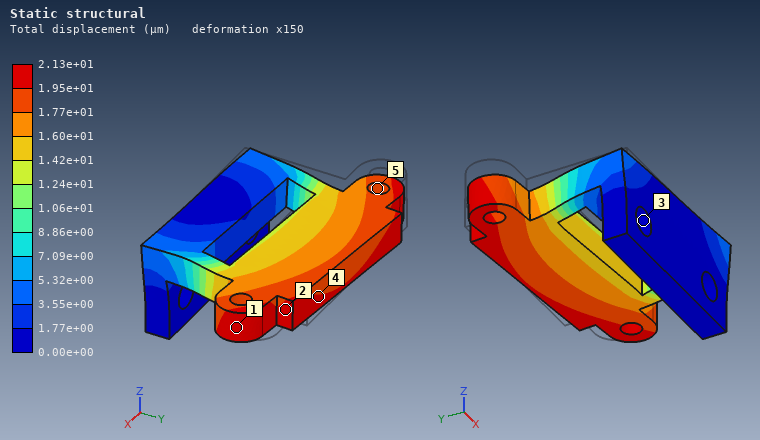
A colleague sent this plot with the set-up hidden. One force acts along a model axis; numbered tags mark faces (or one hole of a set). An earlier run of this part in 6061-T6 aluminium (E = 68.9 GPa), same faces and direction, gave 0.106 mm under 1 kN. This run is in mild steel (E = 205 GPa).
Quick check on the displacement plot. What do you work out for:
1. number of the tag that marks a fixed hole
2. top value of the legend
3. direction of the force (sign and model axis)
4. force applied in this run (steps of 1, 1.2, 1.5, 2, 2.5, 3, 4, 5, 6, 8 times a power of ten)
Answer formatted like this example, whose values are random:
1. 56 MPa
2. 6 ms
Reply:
1. 3
2. 2.13e+01 µm
3. +X
4. 600 N
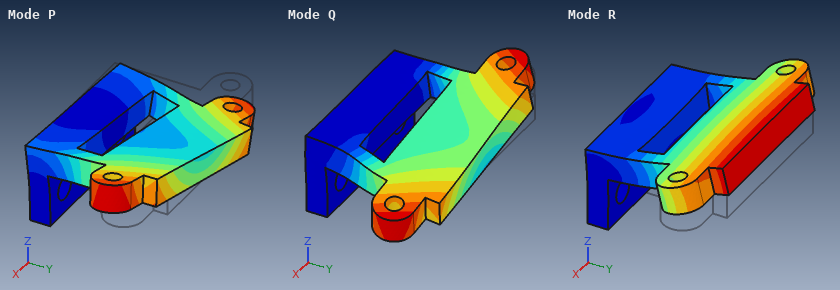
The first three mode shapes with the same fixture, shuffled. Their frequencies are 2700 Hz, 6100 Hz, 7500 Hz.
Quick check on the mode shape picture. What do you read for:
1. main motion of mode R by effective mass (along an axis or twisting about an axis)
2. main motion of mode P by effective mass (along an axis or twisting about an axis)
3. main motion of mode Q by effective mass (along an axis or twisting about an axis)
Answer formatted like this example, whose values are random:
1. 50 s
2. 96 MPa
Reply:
1. along Z
2. along X
3. along X
